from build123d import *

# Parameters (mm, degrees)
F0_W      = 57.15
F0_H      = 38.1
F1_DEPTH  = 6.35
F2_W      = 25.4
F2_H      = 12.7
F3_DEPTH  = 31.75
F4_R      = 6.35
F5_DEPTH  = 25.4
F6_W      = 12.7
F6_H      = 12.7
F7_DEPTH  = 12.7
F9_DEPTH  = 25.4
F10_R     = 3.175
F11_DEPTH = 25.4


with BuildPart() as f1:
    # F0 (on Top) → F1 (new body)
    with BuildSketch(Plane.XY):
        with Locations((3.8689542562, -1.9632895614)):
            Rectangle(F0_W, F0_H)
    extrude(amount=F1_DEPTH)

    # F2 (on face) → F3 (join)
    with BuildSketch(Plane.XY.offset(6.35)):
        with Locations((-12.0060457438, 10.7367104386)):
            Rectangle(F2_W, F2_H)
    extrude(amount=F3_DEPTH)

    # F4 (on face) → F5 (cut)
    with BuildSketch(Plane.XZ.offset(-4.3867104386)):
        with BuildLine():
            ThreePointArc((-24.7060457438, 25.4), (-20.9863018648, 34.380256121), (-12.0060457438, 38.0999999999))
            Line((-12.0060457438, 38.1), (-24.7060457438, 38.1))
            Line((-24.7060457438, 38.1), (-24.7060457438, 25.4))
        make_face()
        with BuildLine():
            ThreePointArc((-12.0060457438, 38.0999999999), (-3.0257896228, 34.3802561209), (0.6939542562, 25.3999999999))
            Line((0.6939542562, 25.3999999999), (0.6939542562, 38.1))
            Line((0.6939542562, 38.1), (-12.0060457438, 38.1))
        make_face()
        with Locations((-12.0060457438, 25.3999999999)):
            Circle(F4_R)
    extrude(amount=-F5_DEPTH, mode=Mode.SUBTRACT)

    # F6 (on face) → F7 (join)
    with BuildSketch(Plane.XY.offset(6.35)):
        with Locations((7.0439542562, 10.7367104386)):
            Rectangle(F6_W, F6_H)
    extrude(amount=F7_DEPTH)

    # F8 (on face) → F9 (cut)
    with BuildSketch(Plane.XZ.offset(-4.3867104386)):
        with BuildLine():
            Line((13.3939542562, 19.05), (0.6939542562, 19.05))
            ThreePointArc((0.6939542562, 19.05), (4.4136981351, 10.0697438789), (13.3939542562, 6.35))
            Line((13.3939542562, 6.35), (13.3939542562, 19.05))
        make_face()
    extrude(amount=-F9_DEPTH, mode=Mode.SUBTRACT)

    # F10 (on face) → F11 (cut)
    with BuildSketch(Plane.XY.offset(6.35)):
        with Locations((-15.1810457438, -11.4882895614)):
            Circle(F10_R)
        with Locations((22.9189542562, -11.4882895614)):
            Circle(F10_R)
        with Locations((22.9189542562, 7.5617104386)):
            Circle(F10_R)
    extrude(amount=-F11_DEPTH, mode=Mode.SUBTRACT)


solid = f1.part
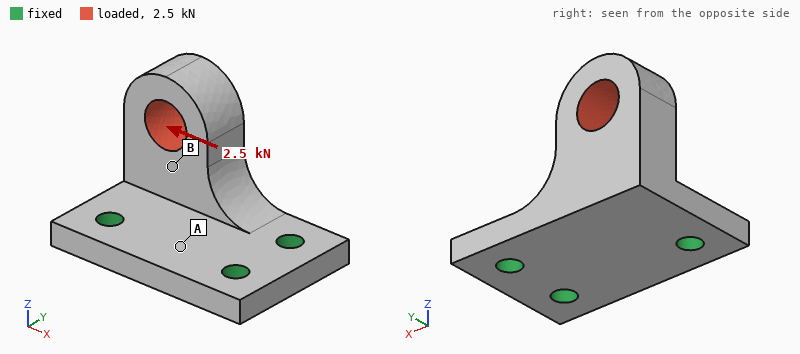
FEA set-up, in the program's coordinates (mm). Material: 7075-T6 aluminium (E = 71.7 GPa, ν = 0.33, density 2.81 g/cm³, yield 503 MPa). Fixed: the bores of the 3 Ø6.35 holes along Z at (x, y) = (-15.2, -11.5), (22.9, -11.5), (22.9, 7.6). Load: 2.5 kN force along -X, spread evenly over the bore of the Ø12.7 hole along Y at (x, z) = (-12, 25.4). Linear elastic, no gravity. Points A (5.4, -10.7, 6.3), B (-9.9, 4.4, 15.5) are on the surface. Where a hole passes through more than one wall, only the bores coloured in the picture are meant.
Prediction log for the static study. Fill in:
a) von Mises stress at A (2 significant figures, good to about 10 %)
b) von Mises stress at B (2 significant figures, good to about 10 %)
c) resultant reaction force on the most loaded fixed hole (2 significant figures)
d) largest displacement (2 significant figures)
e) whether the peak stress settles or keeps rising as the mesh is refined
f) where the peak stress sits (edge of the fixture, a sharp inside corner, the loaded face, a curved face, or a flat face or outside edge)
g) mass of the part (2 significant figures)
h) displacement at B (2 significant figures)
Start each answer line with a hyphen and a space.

- 18 MPa
- 48 MPa
- 1.8 kN
- 0.18 mm
- keeps rising
- edge of the fixture
- 60 g
- 0.065 mm
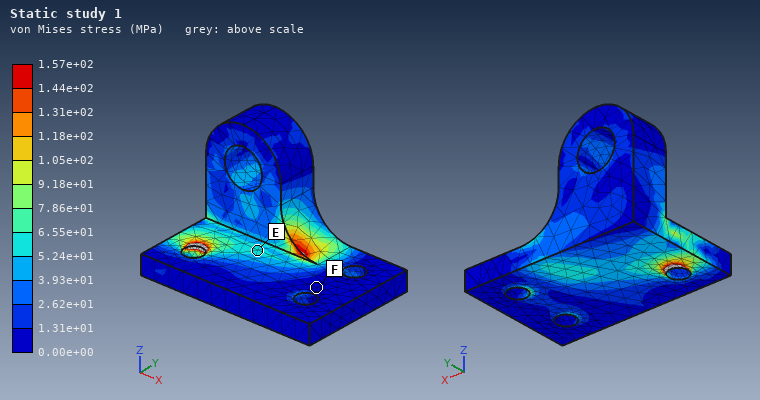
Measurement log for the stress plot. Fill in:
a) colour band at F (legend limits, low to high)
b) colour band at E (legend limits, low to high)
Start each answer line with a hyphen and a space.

- 0.00e+00 to 1.31e+01 MPa
- 5.24e+01 to 6.55e+01 MPa
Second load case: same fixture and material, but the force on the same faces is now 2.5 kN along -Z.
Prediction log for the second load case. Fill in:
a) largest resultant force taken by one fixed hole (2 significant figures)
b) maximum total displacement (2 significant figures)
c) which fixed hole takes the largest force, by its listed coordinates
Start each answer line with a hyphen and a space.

- 1.9 kN
- 0.23 mm
- (-15.2, -11.5)
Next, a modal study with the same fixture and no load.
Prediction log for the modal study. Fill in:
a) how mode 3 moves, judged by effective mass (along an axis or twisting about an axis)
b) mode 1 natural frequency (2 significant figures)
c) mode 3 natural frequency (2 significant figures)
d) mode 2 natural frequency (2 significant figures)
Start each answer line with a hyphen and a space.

- along Z
- 3100 Hz
- 10 kHz
- 6700 Hz
